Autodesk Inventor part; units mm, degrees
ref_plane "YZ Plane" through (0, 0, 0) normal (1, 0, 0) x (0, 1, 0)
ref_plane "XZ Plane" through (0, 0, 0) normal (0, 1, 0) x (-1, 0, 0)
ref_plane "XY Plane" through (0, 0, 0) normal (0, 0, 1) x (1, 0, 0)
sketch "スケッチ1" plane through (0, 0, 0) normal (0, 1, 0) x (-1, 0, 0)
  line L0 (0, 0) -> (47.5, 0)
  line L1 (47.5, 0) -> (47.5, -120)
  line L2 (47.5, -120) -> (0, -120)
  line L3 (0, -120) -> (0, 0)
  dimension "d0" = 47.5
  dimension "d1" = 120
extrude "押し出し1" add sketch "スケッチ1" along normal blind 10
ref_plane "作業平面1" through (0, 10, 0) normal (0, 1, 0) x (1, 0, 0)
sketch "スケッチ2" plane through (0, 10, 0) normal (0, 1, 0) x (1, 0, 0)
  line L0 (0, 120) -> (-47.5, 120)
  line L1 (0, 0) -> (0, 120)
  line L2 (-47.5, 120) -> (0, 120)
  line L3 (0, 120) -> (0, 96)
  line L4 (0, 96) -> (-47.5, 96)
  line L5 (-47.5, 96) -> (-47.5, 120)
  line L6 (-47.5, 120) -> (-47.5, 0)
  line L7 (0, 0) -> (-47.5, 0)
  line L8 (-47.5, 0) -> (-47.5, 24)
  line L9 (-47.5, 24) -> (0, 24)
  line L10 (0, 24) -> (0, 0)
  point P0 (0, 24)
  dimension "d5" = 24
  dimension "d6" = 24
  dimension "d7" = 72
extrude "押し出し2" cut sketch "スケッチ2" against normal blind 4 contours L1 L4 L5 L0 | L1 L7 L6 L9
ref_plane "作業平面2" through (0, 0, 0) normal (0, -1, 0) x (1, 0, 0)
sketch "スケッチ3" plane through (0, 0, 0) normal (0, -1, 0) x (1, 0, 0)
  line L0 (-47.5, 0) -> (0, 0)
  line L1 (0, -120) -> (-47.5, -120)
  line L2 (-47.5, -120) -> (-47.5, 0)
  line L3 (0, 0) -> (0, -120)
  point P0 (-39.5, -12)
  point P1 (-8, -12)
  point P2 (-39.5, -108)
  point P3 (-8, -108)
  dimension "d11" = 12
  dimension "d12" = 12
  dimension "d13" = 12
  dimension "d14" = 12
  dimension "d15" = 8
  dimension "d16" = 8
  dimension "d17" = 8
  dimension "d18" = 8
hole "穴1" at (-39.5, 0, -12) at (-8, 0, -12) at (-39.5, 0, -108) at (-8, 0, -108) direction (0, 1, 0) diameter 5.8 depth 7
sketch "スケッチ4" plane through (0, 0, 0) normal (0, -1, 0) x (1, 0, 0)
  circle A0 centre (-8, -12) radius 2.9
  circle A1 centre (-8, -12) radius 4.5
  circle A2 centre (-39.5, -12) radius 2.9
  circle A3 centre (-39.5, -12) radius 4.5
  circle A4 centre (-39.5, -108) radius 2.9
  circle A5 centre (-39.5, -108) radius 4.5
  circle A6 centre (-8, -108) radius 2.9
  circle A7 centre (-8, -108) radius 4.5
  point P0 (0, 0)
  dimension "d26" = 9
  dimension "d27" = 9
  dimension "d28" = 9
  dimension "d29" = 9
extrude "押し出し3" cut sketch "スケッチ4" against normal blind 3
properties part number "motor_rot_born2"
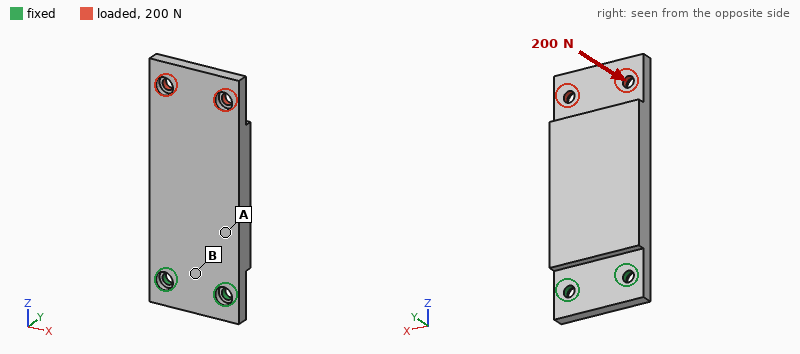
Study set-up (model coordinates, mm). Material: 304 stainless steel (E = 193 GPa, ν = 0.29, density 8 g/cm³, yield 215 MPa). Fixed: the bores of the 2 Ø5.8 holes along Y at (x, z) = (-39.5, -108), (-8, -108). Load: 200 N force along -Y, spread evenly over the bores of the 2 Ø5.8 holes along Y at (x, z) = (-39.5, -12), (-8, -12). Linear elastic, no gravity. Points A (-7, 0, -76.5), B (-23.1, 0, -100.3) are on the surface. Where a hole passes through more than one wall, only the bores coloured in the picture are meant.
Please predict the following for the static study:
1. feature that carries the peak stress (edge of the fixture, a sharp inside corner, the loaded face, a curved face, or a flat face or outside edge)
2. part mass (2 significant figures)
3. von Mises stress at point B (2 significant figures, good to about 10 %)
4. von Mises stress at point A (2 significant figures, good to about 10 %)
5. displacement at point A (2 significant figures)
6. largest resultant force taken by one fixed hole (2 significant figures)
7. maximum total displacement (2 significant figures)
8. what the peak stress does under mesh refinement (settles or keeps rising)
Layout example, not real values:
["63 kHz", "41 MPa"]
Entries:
["edge of the fixture", "370 g", "55 MPa", "16 MPa", "0.069 mm", "120 N", "0.31 mm", "keeps rising"]
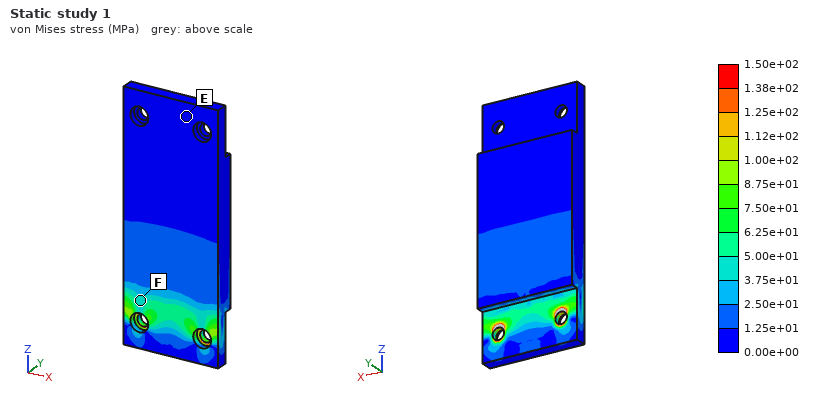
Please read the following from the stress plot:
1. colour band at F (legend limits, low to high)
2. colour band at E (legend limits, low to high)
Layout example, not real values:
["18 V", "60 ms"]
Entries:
["3.75e+01 to 5.00e+01 MPa", "0.00e+00 to 1.25e+01 MPa"]
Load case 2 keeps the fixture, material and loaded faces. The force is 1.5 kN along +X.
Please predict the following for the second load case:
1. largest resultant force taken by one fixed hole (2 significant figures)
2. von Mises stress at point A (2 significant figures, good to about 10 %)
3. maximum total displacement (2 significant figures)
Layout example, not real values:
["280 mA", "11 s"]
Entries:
["4.3 kN", "23 MPa", "58 µm"]
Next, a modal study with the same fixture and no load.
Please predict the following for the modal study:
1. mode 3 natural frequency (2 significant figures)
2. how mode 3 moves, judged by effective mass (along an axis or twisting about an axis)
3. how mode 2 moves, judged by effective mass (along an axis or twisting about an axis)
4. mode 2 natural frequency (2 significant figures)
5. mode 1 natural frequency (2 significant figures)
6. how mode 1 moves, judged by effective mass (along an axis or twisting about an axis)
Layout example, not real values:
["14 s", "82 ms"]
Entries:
["2700 Hz", "twisting about Z", "along X", "2500 Hz", "400 Hz", "along Y"]
